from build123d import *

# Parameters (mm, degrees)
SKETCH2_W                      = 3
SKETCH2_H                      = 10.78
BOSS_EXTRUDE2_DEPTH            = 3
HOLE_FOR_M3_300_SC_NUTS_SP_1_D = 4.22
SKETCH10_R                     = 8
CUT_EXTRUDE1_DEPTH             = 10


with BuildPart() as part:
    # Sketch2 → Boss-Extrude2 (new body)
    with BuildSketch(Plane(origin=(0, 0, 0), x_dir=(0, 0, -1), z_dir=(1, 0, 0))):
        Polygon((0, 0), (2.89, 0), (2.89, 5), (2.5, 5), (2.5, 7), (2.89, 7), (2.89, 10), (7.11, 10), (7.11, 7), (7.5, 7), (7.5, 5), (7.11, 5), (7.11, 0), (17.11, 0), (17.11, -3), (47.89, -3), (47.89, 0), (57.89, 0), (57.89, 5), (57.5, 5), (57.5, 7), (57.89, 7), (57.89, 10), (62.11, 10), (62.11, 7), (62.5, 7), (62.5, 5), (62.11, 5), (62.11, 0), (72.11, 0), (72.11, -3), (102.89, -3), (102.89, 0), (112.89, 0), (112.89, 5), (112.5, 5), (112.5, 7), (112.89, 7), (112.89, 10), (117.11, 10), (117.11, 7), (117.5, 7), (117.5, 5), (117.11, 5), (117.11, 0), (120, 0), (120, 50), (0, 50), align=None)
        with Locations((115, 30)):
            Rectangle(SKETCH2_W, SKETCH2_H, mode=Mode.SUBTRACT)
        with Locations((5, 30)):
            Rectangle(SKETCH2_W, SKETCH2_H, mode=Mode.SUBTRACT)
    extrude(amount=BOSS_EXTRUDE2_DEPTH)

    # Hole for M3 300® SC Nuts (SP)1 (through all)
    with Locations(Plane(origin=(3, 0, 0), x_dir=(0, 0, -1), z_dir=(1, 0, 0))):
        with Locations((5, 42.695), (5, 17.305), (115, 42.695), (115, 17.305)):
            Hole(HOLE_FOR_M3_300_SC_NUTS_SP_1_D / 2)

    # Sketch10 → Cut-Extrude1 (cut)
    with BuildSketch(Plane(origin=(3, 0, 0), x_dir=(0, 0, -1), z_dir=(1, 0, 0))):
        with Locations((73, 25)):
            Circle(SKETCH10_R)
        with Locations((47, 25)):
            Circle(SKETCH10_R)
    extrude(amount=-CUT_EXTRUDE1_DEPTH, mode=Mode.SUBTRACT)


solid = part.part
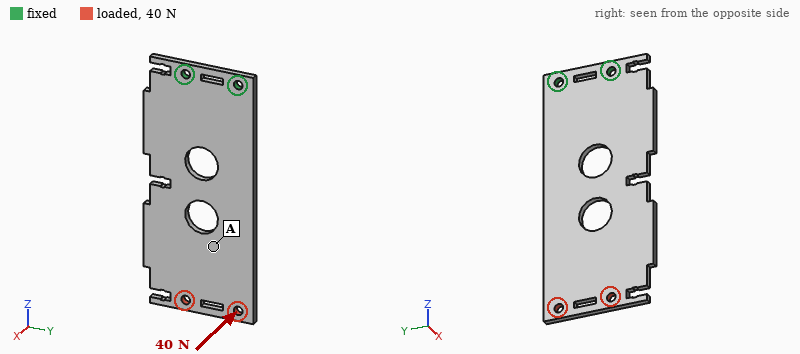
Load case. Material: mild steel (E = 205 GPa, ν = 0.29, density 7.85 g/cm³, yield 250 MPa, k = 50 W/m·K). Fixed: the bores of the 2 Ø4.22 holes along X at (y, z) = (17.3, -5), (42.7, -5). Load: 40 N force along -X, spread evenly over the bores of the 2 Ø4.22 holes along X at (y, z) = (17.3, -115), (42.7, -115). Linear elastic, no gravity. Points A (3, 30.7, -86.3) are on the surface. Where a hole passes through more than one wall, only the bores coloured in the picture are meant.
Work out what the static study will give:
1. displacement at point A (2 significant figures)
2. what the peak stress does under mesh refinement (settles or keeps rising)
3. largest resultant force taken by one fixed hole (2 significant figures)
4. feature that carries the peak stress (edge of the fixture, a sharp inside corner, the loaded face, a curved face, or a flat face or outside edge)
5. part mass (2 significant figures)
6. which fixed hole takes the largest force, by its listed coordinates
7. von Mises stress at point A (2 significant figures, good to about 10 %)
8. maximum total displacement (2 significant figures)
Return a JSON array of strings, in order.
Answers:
["0.56 mm", "keeps rising", "28 N", "edge of the fixture", "130 g", "(17.3, -5)", "13 MPa", "0.99 mm"]
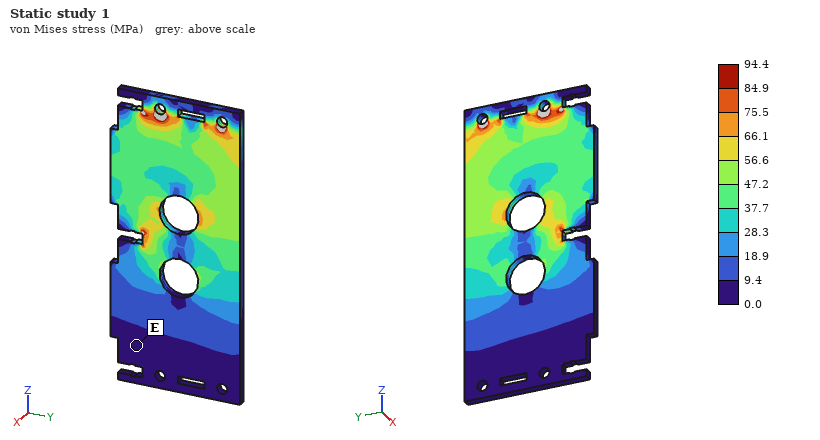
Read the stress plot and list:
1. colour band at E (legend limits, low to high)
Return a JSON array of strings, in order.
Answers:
["0.0 to 9.4 MPa"]
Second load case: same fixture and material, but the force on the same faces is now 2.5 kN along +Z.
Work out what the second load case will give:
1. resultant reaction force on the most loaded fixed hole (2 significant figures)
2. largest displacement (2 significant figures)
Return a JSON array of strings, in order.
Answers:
["1.3 kN", "16 µm"]
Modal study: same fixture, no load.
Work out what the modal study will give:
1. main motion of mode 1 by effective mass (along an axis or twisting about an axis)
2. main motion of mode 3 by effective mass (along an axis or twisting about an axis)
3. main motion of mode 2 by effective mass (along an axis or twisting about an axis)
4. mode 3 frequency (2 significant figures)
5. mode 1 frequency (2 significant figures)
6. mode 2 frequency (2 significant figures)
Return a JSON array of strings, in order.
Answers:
["along X", "along X", "twisting about Z", "1100 Hz", "180 Hz", "790 Hz"]
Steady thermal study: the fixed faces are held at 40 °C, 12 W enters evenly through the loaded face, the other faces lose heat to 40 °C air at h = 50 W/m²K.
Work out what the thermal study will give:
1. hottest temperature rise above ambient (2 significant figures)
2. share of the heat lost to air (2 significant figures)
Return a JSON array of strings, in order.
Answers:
["69 K", "94 %"]
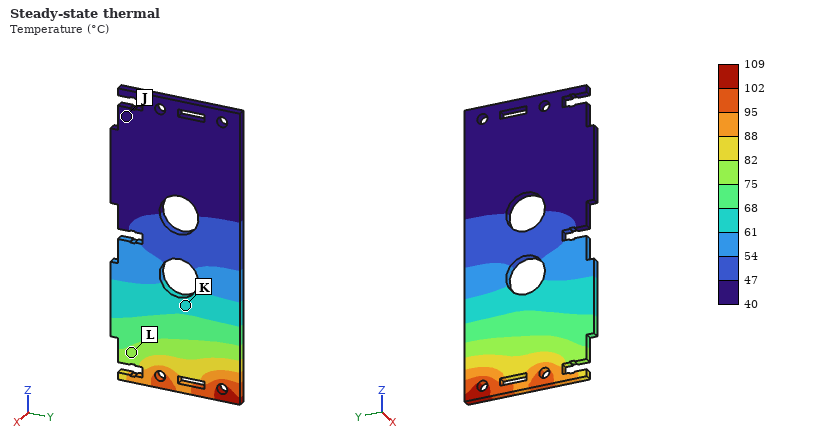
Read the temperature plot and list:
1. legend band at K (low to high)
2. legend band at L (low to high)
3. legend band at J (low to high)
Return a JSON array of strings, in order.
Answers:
["61 to 68 °C", "75 to 82 °C", "40 to 47 °C"]
